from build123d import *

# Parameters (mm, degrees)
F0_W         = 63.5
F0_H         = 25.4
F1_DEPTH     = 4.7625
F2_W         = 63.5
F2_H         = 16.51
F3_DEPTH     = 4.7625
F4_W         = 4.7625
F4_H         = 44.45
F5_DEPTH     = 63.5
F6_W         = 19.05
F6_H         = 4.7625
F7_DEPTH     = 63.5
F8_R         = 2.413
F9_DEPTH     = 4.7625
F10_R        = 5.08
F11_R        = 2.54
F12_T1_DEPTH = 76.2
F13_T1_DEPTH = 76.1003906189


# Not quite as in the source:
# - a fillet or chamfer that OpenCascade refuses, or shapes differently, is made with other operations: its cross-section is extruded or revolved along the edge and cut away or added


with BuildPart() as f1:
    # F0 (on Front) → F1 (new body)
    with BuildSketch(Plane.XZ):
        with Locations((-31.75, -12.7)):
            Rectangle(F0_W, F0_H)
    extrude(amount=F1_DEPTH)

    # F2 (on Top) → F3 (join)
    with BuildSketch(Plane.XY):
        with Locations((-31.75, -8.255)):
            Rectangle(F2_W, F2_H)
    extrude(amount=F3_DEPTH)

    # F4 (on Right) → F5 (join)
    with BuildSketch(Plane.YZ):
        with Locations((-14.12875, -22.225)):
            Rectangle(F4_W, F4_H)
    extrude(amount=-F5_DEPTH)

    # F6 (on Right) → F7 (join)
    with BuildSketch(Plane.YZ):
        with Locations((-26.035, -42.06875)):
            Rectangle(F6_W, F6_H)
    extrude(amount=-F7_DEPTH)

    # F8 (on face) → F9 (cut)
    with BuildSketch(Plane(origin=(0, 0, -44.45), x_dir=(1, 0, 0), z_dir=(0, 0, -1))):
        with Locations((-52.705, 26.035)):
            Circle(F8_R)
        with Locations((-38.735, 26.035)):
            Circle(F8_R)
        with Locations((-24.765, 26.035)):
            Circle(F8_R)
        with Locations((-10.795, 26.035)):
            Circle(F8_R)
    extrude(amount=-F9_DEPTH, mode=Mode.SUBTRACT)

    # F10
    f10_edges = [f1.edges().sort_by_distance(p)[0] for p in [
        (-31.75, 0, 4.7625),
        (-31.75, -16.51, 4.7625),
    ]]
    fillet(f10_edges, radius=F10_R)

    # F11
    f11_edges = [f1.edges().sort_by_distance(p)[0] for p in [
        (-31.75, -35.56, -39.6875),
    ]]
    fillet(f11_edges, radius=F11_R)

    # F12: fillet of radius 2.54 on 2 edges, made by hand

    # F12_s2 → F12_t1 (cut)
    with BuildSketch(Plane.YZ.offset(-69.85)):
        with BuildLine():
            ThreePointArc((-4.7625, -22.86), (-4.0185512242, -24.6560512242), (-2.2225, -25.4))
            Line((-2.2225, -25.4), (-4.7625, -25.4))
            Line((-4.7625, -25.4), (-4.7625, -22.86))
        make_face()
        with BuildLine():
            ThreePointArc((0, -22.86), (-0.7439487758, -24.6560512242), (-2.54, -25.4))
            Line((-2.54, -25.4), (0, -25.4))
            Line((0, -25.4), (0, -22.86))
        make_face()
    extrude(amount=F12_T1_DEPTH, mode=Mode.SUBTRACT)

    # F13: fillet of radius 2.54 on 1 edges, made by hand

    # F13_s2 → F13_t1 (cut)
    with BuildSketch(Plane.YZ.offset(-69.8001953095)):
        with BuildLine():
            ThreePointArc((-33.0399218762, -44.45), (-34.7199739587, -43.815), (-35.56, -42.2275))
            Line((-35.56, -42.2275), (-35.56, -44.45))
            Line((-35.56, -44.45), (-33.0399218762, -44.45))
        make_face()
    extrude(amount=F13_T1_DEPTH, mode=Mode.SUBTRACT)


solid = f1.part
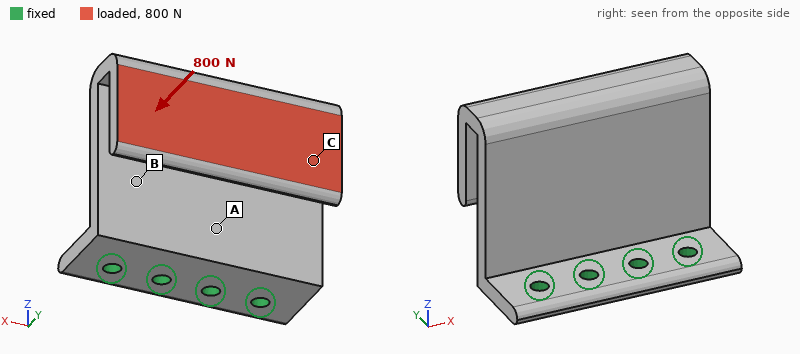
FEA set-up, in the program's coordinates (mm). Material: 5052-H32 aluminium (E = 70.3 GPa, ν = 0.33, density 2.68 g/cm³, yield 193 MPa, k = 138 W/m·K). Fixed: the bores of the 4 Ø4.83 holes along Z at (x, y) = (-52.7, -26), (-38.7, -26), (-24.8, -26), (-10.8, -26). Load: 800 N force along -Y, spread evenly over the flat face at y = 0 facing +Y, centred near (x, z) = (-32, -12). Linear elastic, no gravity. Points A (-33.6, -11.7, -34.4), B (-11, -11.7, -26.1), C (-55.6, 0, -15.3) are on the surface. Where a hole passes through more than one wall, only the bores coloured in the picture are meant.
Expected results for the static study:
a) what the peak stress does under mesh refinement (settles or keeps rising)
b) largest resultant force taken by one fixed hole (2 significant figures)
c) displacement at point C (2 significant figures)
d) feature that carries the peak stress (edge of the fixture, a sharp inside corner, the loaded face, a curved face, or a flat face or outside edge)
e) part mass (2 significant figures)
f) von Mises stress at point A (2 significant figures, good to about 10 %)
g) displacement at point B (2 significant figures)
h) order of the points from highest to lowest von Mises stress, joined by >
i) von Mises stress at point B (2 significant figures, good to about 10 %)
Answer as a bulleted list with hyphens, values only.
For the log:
- keeps rising
- 230 N
- 0.42 mm
- edge of the fixture
- 82 g
- 67 MPa
- 0.16 mm
- A > B > C
- 44 MPa
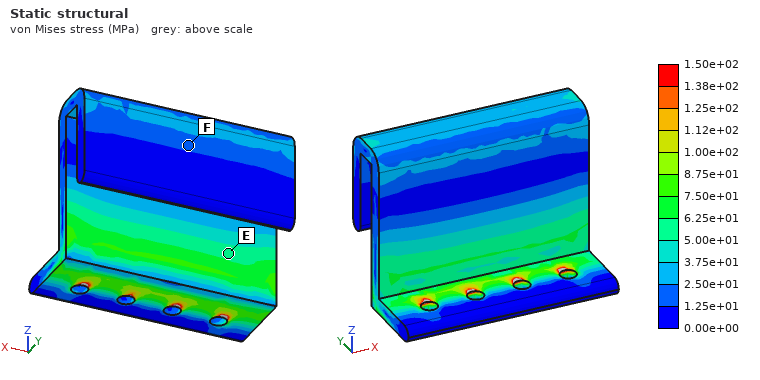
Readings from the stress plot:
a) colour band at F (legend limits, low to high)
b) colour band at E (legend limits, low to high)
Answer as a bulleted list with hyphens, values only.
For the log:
- 1.25e+01 to 2.50e+01 MPa
- 5.00e+01 to 6.25e+01 MPa
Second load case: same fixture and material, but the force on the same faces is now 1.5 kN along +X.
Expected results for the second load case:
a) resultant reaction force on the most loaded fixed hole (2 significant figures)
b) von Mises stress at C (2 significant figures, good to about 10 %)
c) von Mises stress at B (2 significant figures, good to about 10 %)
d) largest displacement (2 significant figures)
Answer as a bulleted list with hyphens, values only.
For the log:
- 1.3 kN
- 11 MPa
- 57 MPa
- 0.35 mm
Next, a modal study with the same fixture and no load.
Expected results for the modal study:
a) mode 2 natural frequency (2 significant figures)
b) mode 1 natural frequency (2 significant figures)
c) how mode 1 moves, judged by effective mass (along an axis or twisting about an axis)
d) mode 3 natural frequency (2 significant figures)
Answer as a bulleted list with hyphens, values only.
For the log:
- 1800 Hz
- 860 Hz
- along Y
- 2500 Hz
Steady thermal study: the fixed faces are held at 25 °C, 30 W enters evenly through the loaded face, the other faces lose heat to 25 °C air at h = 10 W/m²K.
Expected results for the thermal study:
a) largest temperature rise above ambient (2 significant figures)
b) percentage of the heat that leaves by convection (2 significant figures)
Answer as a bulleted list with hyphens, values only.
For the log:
- 50 K
- 10 %
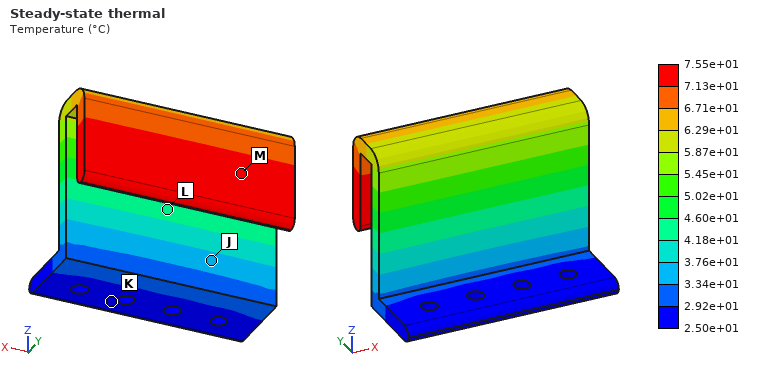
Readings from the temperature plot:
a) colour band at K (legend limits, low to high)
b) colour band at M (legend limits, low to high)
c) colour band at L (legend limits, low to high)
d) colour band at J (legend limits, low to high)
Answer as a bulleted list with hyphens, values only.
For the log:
- 2.50e+01 to 2.92e+01 °C
- 7.13e+01 to 7.55e+01 °C
- 4.18e+01 to 4.60e+01 °C
- 3.34e+01 to 3.76e+01 °C
